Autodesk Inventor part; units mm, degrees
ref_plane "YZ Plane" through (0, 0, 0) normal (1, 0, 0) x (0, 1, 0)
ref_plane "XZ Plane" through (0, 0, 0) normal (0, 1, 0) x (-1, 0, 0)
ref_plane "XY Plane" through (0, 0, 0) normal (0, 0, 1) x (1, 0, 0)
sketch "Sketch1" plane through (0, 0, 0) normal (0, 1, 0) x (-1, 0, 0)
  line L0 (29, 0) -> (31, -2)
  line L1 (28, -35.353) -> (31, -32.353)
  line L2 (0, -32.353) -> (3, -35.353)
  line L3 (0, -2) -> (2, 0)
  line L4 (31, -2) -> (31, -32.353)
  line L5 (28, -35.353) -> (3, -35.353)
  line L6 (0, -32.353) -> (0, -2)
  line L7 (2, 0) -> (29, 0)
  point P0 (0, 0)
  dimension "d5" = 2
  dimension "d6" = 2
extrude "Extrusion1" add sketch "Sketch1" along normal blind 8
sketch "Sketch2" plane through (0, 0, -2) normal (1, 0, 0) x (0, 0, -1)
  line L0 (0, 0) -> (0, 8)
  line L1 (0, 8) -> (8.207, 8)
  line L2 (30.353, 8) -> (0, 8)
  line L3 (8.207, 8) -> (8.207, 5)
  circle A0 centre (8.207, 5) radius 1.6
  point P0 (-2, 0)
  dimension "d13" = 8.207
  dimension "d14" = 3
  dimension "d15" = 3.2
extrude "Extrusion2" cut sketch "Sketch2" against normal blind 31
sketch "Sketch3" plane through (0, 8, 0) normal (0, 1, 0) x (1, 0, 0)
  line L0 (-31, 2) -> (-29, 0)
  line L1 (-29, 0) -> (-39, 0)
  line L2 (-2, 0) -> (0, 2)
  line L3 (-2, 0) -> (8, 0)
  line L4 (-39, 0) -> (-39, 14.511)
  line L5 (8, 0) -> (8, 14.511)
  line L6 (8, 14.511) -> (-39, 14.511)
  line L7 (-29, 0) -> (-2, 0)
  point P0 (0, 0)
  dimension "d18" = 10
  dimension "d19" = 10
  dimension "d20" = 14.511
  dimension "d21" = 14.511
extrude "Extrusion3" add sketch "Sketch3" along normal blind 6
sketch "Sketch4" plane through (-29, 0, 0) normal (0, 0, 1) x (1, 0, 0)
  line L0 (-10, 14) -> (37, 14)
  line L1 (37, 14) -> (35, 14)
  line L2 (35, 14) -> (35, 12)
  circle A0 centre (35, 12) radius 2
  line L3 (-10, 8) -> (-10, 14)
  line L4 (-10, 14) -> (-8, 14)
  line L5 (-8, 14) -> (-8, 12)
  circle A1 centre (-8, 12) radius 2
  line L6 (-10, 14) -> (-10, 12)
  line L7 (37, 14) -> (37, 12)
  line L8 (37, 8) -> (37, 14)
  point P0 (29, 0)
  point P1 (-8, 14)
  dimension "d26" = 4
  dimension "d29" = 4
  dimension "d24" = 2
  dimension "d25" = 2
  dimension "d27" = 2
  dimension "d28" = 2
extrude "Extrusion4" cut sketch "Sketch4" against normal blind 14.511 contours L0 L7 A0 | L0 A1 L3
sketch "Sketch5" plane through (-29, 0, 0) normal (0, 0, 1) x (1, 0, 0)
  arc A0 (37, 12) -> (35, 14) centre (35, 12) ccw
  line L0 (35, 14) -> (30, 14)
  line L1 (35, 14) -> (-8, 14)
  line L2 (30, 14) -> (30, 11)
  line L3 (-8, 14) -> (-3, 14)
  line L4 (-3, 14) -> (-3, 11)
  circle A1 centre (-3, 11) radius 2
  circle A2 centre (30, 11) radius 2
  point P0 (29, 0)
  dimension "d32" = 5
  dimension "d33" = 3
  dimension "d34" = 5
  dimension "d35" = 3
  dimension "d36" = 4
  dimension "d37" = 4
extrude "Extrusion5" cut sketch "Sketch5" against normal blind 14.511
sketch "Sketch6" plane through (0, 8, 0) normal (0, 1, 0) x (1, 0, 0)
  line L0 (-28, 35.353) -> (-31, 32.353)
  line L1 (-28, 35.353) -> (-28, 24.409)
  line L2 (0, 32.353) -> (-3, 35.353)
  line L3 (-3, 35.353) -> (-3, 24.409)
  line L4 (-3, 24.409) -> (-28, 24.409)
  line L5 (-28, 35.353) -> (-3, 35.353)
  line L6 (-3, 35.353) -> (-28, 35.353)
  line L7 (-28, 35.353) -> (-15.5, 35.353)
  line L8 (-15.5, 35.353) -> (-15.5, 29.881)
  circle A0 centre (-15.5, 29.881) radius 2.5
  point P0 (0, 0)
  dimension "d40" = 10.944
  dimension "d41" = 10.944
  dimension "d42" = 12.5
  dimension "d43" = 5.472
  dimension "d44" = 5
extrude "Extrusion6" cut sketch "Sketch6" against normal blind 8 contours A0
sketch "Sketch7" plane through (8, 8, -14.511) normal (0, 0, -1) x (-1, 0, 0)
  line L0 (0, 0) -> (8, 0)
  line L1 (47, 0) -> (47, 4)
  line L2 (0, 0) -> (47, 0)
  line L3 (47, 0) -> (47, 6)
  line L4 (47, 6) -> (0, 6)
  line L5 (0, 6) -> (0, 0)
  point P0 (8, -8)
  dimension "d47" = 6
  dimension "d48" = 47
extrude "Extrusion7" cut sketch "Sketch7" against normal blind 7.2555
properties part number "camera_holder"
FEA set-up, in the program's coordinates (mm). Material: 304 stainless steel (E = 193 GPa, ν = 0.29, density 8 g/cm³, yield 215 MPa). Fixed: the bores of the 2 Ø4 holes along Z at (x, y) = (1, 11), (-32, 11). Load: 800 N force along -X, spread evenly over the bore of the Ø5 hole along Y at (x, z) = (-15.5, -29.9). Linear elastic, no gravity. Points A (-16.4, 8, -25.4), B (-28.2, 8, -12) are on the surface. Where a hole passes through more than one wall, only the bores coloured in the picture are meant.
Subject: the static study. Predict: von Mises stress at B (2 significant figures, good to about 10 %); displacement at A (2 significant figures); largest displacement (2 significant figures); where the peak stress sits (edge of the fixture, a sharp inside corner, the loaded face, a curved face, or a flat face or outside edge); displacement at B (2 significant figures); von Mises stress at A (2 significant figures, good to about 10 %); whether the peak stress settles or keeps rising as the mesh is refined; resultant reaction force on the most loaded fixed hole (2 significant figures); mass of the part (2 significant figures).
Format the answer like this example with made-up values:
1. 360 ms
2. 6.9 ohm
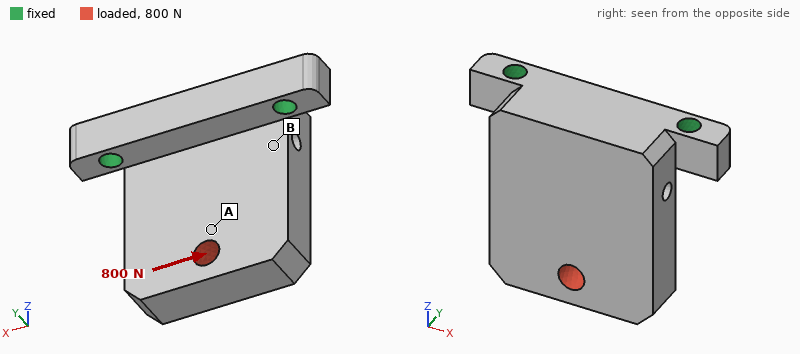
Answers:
1. 30 MPa
2. 6.0 µm
3. 9.2 µm
4. a sharp inside corner
5. 3.1 µm
6. 13 MPa
7. keeps rising
8. 850 N
9. 81 g
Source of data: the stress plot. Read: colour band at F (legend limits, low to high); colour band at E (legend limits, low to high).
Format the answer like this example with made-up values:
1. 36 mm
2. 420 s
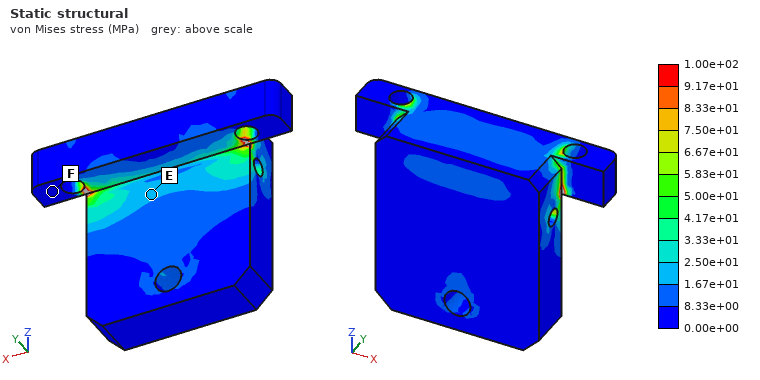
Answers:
1. 0.00e+00 to 8.33e+00 MPa
2. 1.67e+01 to 2.50e+01 MPa
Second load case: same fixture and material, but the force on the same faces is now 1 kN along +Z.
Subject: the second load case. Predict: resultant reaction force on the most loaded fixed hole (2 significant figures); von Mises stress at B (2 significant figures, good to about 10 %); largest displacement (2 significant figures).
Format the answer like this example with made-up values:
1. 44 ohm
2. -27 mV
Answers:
1. 500 N
2. 13 MPa
3. 15 µm
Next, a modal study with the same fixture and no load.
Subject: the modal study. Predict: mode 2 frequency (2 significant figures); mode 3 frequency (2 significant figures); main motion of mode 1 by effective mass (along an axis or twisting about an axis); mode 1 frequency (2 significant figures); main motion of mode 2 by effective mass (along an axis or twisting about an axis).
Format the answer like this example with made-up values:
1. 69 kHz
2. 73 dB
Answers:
1. 9200 Hz
2. 13 kHz
3. along Y
4. 3300 Hz
5. along X
